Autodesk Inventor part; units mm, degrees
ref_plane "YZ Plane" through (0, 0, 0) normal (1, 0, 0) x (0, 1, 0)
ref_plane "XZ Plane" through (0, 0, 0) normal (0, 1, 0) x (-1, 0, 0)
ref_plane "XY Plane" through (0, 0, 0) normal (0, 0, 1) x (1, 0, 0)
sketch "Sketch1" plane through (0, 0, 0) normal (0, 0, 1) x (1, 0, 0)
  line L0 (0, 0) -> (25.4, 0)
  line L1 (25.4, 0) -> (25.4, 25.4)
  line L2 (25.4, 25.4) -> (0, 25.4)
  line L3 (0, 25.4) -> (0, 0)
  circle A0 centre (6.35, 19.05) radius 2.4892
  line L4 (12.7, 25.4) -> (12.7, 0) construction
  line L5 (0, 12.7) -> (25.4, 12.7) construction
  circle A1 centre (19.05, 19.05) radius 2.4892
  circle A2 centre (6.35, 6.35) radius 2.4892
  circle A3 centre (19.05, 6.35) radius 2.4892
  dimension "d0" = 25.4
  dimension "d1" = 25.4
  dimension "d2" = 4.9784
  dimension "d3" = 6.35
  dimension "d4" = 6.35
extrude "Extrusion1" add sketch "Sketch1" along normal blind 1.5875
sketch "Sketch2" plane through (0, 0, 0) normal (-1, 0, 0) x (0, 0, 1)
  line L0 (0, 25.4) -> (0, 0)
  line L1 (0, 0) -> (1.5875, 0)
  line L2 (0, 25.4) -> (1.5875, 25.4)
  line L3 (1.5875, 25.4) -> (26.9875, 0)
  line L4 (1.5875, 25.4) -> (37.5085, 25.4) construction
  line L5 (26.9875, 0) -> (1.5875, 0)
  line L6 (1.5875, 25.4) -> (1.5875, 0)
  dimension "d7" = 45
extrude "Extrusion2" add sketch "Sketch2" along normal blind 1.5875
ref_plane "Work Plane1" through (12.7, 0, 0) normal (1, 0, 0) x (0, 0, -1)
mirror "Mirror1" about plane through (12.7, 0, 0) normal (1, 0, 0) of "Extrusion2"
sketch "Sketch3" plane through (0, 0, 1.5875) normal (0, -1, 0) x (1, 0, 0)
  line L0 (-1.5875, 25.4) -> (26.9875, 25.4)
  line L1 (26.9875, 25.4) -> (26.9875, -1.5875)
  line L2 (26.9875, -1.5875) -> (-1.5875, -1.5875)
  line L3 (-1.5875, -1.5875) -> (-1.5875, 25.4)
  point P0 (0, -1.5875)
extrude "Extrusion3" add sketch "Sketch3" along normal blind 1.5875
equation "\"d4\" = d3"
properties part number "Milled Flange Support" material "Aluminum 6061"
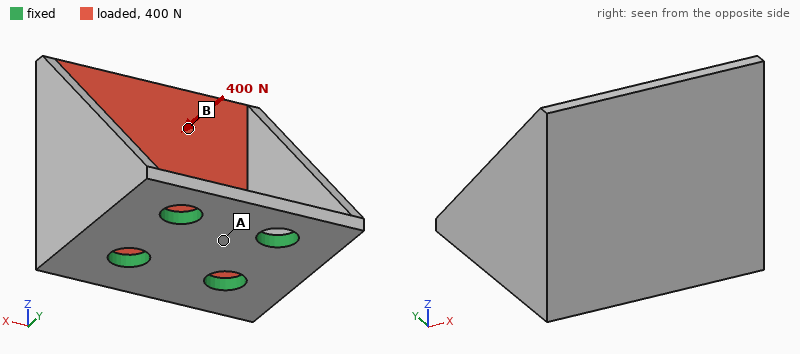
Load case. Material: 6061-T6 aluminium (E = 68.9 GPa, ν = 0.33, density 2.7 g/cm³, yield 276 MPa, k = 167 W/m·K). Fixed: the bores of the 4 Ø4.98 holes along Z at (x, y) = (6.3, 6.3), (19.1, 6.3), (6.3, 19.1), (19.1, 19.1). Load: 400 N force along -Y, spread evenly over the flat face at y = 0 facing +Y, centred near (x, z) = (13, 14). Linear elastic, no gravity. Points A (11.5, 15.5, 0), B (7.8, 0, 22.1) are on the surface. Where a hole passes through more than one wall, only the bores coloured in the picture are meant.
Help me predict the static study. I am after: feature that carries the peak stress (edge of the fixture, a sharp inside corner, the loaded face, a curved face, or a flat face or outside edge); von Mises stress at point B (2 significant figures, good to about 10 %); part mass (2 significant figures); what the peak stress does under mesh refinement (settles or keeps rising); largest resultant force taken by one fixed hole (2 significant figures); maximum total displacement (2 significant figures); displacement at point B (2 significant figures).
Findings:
edge of the fixture
59 MPa
8.8 g
keeps rising
210 N
0.18 mm
0.13 mm
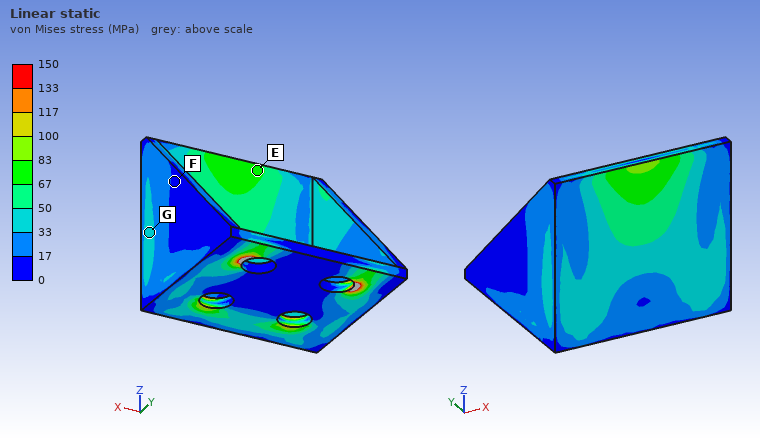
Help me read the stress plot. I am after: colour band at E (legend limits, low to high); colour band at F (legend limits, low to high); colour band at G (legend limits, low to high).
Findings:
67 to 83 MPa
0 to 17 MPa
33 to 50 MPa
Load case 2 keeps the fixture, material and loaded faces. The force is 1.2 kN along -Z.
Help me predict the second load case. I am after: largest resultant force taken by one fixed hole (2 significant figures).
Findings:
700 N
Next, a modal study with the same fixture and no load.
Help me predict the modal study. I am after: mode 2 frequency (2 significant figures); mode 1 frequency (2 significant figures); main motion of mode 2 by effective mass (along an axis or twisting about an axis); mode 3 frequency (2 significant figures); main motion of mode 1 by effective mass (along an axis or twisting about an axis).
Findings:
5100 Hz
4900 Hz
along Y
9600 Hz
along X
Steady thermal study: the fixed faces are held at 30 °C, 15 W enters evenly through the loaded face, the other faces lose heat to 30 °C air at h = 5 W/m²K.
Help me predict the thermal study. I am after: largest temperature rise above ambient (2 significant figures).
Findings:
24 K
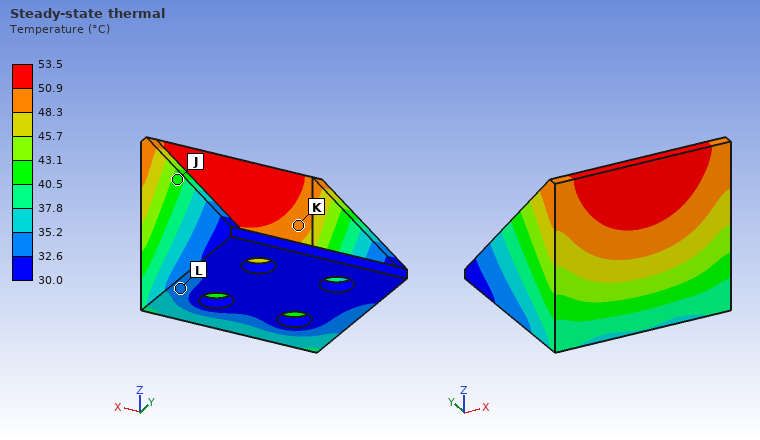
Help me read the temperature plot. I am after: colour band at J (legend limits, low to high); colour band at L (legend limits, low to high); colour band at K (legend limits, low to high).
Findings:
40.5 to 43.1 °C
32.6 to 35.2 °C
48.3 to 50.9 °C
